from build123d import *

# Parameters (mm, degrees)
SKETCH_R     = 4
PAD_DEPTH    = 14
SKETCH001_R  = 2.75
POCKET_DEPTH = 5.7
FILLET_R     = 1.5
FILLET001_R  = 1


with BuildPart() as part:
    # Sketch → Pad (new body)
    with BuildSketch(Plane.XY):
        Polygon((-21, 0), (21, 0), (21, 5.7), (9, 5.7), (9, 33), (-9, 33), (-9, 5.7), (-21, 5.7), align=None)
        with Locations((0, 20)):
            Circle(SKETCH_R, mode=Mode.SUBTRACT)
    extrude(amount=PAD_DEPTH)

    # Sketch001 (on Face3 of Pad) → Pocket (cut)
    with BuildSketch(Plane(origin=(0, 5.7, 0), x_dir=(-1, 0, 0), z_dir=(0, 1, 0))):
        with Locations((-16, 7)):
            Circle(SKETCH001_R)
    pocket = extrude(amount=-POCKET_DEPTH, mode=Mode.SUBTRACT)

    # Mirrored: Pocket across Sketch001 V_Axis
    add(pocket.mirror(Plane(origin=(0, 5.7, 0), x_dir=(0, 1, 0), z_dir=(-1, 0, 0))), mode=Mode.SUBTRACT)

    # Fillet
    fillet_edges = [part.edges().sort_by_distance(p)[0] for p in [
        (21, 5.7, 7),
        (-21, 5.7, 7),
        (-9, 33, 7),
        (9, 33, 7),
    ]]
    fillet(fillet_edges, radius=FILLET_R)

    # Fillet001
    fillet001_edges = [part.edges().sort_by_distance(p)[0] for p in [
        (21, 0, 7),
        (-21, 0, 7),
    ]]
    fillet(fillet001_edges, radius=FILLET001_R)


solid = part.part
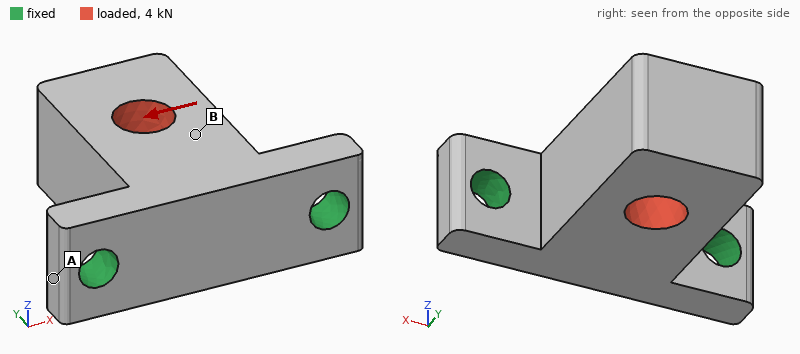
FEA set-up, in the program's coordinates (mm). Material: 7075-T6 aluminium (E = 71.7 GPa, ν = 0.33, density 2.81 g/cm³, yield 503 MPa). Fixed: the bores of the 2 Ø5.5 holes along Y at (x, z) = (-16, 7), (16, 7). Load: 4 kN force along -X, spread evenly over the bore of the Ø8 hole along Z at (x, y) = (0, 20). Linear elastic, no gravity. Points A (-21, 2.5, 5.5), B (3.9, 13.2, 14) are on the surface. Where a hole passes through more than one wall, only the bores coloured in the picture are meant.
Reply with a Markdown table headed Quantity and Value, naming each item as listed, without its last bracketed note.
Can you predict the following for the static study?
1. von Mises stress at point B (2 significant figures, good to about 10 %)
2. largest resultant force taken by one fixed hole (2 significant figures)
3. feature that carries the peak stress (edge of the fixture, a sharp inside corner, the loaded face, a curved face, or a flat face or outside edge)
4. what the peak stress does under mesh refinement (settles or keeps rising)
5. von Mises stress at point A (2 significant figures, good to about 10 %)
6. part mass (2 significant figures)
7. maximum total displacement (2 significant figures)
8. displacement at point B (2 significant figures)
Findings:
| Quantity | Value |
|---|---|
| von Mises stress at point B | 31 MPa |
| largest resultant force taken by one fixed hole | 3.5 kN |
| feature that carries the peak stress | edge of the fixture |
| what the peak stress does under mesh refinement | keeps rising |
| von Mises stress at point A | 16 MPa |
| part mass | 26 g |
| maximum total displacement | 90 µm |
| displacement at point B | 26 µm |
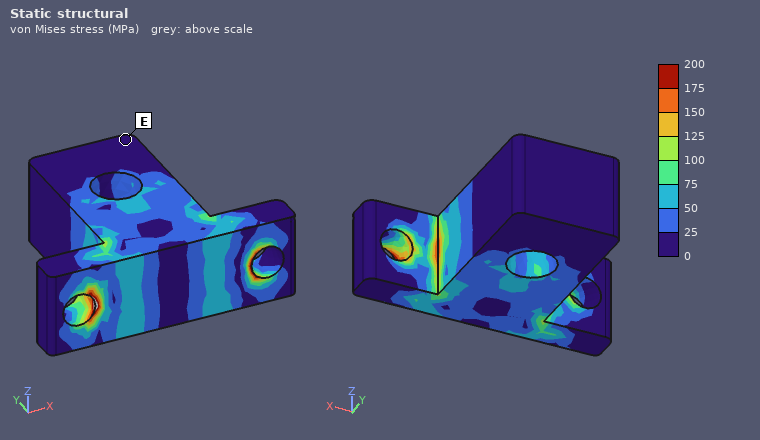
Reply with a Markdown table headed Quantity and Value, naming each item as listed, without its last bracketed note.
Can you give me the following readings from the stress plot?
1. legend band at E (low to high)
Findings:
| Quantity | Value |
|---|---|
| legend band at E | 0 to 25 MPa |
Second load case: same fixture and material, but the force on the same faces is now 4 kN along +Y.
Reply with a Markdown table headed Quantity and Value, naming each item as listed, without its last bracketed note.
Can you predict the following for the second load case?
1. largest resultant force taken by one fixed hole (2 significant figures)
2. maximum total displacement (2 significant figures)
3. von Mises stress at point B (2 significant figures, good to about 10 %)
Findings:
| Quantity | Value |
|---|---|
| largest resultant force taken by one fixed hole | 2.1 kN |
| maximum total displacement | 20 µm |
| von Mises stress at point B | 16 MPa |
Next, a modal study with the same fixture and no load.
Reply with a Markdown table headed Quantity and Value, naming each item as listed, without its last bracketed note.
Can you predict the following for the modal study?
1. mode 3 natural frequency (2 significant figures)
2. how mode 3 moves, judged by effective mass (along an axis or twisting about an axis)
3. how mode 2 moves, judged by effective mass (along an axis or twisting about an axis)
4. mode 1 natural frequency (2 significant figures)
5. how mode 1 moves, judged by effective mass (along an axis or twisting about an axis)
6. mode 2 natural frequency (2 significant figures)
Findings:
| Quantity | Value |
|---|---|
| mode 3 natural frequency | 17 kHz |
| how mode 3 moves, judged by effective mass | along Y |
| how mode 2 moves, judged by effective mass | along X |
| mode 1 natural frequency | 4600 Hz |
| how mode 1 moves, judged by effective mass | along Z |
| mode 2 natural frequency | 9500 Hz |
